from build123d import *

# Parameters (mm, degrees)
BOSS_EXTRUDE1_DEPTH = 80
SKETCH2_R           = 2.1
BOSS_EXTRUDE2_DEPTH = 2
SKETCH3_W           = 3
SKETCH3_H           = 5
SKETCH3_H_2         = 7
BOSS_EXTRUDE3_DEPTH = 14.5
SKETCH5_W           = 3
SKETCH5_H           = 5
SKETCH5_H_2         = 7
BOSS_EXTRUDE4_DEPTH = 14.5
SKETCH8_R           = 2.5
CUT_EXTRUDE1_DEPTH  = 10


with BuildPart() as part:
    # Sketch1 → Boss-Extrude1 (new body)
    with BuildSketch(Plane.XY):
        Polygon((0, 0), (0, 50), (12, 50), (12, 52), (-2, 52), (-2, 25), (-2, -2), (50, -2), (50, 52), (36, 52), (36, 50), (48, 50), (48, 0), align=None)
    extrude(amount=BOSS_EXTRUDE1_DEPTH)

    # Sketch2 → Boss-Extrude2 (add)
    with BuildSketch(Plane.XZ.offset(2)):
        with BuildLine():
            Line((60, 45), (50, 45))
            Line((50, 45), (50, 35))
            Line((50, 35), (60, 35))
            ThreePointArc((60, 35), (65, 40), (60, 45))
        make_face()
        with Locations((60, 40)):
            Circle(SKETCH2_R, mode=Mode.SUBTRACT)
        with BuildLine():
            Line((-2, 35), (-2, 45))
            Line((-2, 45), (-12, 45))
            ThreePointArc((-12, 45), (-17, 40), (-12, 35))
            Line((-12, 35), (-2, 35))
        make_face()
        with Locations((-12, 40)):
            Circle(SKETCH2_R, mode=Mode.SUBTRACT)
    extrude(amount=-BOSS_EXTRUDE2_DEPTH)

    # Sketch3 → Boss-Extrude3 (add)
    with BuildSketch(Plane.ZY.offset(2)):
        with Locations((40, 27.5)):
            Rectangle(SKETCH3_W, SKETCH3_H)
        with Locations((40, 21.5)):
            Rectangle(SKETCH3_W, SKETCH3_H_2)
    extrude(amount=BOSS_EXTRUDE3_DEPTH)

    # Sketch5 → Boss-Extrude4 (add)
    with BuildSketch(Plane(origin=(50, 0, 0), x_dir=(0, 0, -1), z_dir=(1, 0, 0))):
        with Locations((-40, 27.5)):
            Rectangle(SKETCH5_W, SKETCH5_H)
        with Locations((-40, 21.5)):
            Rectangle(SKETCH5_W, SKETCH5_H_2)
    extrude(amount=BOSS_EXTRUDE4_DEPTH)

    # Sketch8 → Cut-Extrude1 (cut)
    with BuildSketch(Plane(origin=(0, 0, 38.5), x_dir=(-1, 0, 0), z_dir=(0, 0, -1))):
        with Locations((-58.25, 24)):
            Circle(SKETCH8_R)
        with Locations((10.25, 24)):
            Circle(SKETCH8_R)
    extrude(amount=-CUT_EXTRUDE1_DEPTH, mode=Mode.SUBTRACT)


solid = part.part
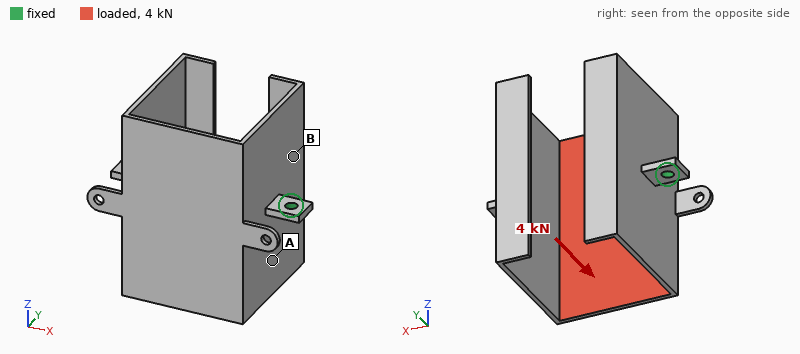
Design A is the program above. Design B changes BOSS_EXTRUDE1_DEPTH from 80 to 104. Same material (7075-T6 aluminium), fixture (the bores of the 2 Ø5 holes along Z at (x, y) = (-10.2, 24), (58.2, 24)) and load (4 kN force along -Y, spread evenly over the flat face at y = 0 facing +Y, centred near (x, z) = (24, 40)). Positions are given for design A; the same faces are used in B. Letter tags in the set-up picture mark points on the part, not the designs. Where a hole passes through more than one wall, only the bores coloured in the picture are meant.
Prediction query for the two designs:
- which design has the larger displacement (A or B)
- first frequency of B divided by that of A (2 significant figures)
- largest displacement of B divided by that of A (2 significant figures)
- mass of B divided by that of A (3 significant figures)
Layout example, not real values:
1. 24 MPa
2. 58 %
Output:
1. B
2. 0.71
3. 4.9
4. 1.29
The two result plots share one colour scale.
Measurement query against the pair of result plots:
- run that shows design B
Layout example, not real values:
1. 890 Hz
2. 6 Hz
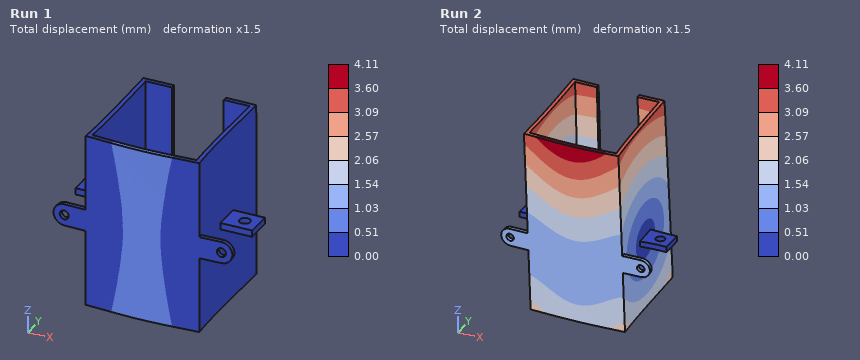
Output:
1. Run 2
